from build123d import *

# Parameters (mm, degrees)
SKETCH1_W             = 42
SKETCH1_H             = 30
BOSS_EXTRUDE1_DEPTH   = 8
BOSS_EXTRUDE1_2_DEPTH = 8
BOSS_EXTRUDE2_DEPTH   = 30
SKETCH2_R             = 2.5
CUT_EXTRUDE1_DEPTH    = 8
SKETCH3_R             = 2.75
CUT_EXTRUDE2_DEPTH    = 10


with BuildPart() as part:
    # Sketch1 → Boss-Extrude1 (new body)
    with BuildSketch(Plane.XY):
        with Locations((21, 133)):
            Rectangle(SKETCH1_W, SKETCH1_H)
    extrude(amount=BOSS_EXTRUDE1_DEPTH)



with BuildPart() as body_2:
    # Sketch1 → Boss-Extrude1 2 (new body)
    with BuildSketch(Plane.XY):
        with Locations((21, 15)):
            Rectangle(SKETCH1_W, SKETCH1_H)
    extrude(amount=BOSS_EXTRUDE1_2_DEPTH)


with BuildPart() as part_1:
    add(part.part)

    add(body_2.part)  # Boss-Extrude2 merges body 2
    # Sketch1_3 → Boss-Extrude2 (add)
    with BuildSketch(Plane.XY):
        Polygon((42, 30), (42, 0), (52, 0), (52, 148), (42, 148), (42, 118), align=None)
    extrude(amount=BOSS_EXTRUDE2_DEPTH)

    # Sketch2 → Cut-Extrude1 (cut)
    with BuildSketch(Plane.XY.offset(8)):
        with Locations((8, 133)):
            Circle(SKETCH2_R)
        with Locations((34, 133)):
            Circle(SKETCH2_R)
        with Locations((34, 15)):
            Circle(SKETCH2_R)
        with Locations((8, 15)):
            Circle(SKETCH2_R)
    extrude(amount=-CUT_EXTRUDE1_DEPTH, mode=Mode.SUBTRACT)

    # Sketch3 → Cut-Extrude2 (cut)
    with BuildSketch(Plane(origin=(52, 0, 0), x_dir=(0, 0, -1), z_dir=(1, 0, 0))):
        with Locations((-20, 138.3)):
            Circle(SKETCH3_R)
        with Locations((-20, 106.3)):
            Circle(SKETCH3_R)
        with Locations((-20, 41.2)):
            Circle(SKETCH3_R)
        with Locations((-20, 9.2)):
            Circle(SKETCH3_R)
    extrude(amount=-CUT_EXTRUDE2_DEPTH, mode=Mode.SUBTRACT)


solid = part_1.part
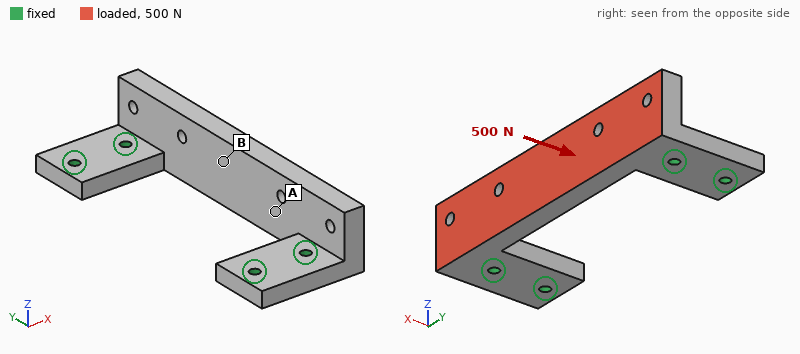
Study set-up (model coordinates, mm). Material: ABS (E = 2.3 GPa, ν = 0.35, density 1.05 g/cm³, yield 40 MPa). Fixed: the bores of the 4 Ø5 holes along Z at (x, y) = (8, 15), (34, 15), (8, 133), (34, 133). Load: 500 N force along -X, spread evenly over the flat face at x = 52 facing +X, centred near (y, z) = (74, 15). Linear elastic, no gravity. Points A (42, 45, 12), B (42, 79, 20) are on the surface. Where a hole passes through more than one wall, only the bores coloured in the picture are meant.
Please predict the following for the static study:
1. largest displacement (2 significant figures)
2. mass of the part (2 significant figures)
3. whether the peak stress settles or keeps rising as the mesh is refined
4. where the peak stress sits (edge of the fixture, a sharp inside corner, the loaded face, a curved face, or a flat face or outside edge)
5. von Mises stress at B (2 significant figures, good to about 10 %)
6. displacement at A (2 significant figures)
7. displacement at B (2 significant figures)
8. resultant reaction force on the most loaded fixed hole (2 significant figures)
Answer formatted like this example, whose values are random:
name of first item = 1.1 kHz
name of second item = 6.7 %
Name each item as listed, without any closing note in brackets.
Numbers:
largest displacement = 0.69 mm
mass of the part = 66 g
whether the peak stress settles or keeps rising as the mesh is refined = keeps rising
where the peak stress sits = edge of the fixture
von Mises stress at B = 3.4 MPa
displacement at A = 0.26 mm
displacement at B = 0.50 mm
resultant reaction force on the most loaded fixed hole = 200 N
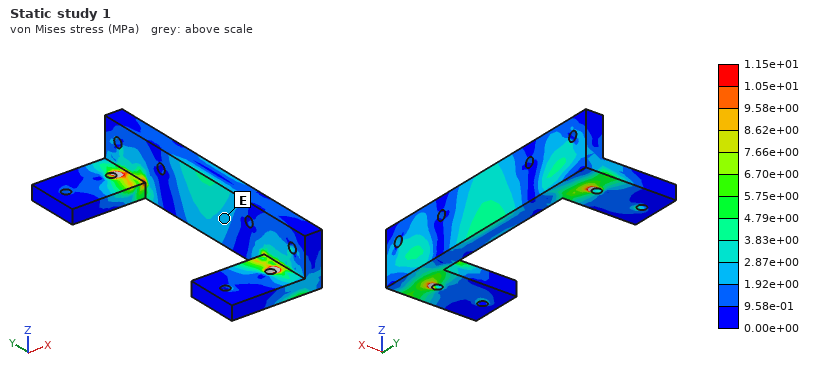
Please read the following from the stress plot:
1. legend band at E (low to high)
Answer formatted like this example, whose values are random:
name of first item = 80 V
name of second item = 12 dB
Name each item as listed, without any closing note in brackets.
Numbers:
legend band at E = 1.92e+00 to 2.87e+00 MPa
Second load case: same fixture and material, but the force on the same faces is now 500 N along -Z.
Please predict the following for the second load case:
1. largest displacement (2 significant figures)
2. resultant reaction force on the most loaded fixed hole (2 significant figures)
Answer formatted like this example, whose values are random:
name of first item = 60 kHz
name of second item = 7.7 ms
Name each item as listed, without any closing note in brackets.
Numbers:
largest displacement = 0.59 mm
resultant reaction force on the most loaded fixed hole = 340 N
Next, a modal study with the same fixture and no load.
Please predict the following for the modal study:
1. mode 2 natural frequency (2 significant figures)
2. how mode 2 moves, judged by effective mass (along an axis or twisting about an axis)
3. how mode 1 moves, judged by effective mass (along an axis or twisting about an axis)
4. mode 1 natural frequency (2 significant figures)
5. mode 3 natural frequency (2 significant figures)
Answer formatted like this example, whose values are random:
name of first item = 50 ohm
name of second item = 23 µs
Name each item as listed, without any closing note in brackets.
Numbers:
mode 2 natural frequency = 1400 Hz
how mode 2 moves, judged by effective mass = along Z
how mode 1 moves, judged by effective mass = along X
mode 1 natural frequency = 790 Hz
mode 3 natural frequency = 1500 Hz
